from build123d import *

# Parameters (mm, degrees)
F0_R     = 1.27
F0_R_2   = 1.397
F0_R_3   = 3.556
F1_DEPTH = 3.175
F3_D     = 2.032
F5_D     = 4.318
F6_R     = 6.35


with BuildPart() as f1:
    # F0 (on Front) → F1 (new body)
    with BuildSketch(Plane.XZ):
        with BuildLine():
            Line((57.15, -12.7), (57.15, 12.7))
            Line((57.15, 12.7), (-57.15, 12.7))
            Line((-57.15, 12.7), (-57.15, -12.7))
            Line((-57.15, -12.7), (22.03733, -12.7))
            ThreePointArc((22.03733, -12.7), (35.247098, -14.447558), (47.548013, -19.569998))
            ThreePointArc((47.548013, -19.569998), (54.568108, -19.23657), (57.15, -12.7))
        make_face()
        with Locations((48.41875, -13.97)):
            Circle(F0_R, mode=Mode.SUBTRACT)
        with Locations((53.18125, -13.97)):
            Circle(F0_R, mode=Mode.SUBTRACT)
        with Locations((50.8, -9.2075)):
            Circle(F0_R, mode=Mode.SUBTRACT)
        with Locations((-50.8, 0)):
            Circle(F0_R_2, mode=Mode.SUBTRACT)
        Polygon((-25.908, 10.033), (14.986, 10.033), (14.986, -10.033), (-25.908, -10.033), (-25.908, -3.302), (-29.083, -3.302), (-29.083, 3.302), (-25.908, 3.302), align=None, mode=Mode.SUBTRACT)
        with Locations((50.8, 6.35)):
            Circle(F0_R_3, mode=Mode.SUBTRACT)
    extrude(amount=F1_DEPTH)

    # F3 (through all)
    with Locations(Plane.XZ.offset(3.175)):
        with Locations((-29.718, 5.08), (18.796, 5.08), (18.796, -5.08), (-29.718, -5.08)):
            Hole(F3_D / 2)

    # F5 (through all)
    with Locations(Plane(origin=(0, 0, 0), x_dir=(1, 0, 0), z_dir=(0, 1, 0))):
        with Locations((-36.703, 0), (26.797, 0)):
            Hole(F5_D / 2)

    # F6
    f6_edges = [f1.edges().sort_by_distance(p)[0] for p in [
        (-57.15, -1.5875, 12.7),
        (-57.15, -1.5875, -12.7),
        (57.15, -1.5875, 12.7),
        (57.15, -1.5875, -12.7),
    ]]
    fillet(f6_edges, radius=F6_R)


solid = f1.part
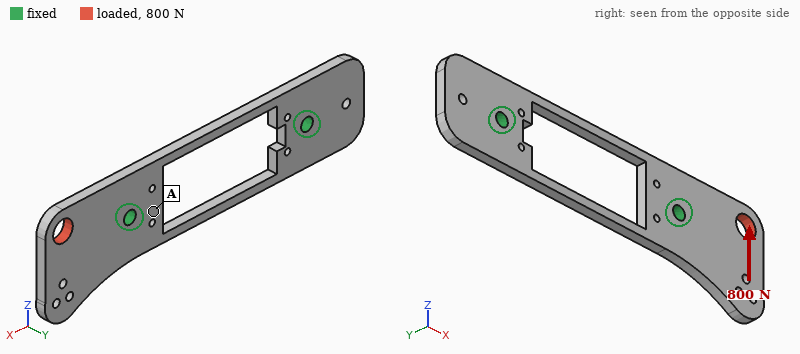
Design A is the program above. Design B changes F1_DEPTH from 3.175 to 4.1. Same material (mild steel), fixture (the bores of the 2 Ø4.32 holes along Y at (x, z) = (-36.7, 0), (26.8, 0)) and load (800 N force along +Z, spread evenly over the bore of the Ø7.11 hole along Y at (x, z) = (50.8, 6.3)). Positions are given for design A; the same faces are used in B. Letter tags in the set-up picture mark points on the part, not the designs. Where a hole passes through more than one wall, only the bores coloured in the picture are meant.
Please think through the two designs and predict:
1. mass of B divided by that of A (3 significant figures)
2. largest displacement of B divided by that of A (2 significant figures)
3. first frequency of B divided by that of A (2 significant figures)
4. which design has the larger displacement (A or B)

1.29
0.77
1.3
A
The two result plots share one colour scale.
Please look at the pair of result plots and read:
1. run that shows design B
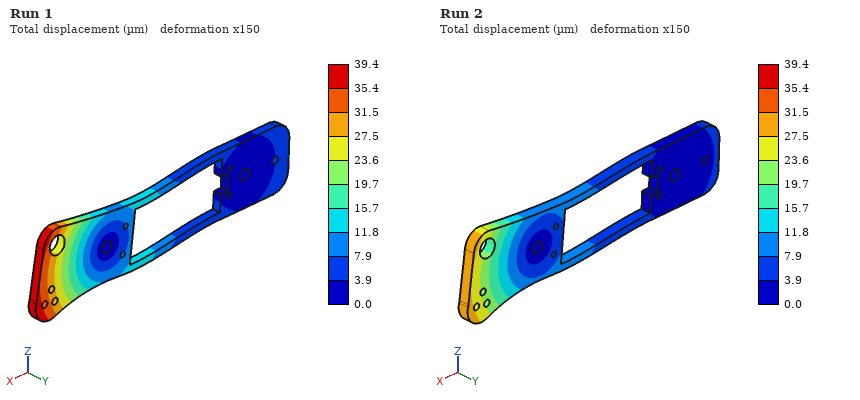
Run 2
